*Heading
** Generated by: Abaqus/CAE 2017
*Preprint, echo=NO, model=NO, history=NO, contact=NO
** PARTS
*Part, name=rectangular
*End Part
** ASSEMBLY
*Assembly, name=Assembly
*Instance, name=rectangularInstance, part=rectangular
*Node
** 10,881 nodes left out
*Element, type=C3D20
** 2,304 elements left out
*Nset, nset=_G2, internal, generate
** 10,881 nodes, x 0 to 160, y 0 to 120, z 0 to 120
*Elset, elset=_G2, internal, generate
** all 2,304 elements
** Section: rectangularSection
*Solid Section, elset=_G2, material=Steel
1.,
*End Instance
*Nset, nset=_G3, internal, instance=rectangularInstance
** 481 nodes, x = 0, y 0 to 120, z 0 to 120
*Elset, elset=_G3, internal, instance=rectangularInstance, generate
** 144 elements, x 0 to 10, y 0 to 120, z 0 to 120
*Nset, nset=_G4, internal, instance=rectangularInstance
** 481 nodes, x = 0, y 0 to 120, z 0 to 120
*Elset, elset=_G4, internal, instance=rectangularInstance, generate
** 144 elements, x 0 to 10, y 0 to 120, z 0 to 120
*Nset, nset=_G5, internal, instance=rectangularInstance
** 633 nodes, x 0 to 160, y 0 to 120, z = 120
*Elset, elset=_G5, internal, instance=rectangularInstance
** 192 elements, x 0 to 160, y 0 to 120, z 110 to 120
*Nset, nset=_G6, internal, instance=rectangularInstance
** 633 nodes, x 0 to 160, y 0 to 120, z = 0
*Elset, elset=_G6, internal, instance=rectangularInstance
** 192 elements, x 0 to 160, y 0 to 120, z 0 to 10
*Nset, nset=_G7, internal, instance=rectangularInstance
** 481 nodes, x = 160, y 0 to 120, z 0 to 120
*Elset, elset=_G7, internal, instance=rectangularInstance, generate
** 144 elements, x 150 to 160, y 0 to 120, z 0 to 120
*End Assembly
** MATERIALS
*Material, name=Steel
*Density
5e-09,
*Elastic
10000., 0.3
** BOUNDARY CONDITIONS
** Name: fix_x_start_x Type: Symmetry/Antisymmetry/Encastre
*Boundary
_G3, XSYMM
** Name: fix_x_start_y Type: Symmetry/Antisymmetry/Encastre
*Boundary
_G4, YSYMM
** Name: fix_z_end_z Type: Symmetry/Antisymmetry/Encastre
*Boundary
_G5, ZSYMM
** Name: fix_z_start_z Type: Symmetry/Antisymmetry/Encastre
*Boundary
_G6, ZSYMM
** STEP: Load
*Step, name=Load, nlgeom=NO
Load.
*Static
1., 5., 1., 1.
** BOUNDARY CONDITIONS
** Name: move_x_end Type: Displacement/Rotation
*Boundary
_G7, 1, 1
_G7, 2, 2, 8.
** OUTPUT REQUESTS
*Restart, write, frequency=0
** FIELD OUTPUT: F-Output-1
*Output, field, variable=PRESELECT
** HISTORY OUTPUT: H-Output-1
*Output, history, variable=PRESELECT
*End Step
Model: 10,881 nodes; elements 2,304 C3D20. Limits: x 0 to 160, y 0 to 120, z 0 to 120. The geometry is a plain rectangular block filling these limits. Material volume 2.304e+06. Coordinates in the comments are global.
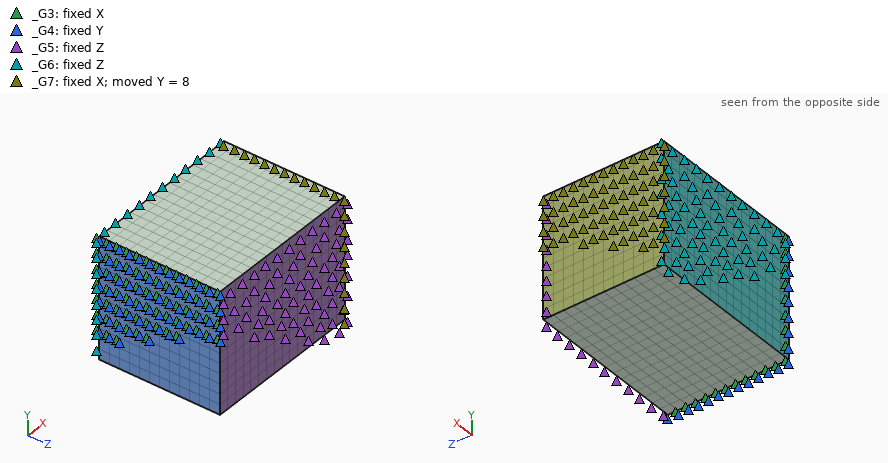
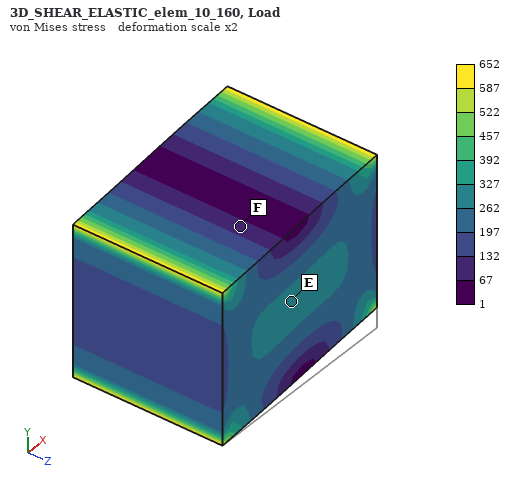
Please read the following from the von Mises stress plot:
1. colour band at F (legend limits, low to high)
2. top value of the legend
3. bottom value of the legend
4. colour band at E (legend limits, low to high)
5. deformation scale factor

67 to 132
652
1
262 to 327
2
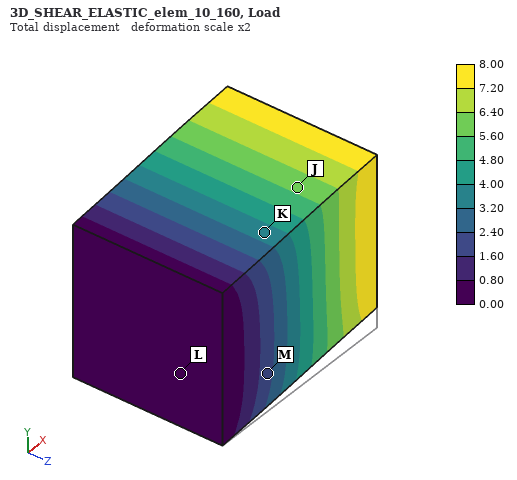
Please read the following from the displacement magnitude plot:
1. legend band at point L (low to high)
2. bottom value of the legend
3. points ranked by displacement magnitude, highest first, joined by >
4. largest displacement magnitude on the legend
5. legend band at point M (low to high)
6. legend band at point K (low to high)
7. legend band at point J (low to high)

0.00 to 0.80
0.00
J > K > M > L
8.00
1.60 to 2.40
3.20 to 4.00
5.60 to 6.40
